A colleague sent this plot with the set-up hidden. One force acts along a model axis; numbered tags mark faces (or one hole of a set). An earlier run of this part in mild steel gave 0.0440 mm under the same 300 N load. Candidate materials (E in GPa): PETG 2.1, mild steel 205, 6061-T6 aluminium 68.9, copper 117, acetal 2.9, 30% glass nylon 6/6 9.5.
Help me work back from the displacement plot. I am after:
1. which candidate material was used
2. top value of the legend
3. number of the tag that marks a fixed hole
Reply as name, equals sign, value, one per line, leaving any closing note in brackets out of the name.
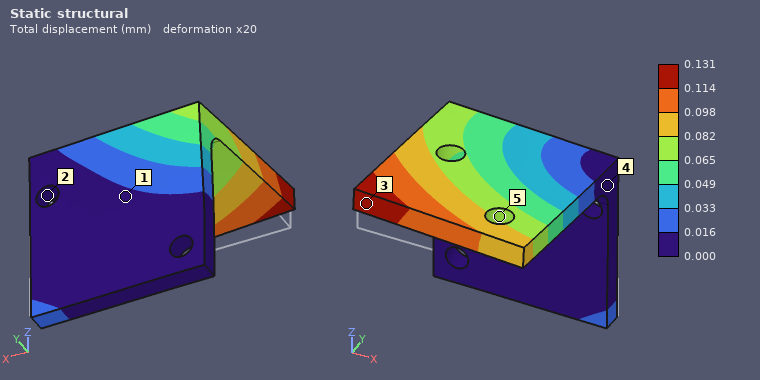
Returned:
which candidate material was used = 6061-T6 aluminium
top value of the legend = 0.131 mm
number of the tag that marks a fixed hole = 2
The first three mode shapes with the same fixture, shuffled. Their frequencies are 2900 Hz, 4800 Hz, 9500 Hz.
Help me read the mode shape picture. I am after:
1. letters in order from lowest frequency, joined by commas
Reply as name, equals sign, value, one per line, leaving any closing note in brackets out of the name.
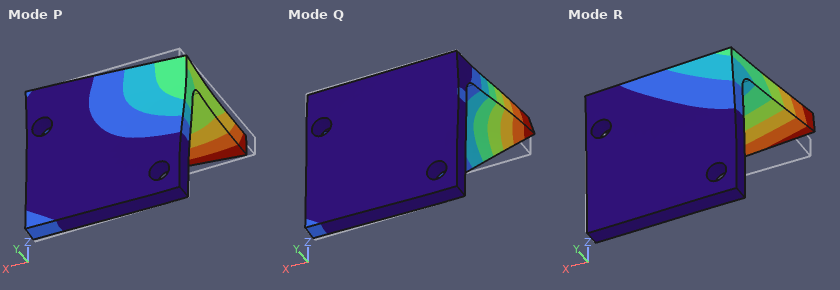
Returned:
letters in order from lowest frequency, joined by commas = R, P, Q
